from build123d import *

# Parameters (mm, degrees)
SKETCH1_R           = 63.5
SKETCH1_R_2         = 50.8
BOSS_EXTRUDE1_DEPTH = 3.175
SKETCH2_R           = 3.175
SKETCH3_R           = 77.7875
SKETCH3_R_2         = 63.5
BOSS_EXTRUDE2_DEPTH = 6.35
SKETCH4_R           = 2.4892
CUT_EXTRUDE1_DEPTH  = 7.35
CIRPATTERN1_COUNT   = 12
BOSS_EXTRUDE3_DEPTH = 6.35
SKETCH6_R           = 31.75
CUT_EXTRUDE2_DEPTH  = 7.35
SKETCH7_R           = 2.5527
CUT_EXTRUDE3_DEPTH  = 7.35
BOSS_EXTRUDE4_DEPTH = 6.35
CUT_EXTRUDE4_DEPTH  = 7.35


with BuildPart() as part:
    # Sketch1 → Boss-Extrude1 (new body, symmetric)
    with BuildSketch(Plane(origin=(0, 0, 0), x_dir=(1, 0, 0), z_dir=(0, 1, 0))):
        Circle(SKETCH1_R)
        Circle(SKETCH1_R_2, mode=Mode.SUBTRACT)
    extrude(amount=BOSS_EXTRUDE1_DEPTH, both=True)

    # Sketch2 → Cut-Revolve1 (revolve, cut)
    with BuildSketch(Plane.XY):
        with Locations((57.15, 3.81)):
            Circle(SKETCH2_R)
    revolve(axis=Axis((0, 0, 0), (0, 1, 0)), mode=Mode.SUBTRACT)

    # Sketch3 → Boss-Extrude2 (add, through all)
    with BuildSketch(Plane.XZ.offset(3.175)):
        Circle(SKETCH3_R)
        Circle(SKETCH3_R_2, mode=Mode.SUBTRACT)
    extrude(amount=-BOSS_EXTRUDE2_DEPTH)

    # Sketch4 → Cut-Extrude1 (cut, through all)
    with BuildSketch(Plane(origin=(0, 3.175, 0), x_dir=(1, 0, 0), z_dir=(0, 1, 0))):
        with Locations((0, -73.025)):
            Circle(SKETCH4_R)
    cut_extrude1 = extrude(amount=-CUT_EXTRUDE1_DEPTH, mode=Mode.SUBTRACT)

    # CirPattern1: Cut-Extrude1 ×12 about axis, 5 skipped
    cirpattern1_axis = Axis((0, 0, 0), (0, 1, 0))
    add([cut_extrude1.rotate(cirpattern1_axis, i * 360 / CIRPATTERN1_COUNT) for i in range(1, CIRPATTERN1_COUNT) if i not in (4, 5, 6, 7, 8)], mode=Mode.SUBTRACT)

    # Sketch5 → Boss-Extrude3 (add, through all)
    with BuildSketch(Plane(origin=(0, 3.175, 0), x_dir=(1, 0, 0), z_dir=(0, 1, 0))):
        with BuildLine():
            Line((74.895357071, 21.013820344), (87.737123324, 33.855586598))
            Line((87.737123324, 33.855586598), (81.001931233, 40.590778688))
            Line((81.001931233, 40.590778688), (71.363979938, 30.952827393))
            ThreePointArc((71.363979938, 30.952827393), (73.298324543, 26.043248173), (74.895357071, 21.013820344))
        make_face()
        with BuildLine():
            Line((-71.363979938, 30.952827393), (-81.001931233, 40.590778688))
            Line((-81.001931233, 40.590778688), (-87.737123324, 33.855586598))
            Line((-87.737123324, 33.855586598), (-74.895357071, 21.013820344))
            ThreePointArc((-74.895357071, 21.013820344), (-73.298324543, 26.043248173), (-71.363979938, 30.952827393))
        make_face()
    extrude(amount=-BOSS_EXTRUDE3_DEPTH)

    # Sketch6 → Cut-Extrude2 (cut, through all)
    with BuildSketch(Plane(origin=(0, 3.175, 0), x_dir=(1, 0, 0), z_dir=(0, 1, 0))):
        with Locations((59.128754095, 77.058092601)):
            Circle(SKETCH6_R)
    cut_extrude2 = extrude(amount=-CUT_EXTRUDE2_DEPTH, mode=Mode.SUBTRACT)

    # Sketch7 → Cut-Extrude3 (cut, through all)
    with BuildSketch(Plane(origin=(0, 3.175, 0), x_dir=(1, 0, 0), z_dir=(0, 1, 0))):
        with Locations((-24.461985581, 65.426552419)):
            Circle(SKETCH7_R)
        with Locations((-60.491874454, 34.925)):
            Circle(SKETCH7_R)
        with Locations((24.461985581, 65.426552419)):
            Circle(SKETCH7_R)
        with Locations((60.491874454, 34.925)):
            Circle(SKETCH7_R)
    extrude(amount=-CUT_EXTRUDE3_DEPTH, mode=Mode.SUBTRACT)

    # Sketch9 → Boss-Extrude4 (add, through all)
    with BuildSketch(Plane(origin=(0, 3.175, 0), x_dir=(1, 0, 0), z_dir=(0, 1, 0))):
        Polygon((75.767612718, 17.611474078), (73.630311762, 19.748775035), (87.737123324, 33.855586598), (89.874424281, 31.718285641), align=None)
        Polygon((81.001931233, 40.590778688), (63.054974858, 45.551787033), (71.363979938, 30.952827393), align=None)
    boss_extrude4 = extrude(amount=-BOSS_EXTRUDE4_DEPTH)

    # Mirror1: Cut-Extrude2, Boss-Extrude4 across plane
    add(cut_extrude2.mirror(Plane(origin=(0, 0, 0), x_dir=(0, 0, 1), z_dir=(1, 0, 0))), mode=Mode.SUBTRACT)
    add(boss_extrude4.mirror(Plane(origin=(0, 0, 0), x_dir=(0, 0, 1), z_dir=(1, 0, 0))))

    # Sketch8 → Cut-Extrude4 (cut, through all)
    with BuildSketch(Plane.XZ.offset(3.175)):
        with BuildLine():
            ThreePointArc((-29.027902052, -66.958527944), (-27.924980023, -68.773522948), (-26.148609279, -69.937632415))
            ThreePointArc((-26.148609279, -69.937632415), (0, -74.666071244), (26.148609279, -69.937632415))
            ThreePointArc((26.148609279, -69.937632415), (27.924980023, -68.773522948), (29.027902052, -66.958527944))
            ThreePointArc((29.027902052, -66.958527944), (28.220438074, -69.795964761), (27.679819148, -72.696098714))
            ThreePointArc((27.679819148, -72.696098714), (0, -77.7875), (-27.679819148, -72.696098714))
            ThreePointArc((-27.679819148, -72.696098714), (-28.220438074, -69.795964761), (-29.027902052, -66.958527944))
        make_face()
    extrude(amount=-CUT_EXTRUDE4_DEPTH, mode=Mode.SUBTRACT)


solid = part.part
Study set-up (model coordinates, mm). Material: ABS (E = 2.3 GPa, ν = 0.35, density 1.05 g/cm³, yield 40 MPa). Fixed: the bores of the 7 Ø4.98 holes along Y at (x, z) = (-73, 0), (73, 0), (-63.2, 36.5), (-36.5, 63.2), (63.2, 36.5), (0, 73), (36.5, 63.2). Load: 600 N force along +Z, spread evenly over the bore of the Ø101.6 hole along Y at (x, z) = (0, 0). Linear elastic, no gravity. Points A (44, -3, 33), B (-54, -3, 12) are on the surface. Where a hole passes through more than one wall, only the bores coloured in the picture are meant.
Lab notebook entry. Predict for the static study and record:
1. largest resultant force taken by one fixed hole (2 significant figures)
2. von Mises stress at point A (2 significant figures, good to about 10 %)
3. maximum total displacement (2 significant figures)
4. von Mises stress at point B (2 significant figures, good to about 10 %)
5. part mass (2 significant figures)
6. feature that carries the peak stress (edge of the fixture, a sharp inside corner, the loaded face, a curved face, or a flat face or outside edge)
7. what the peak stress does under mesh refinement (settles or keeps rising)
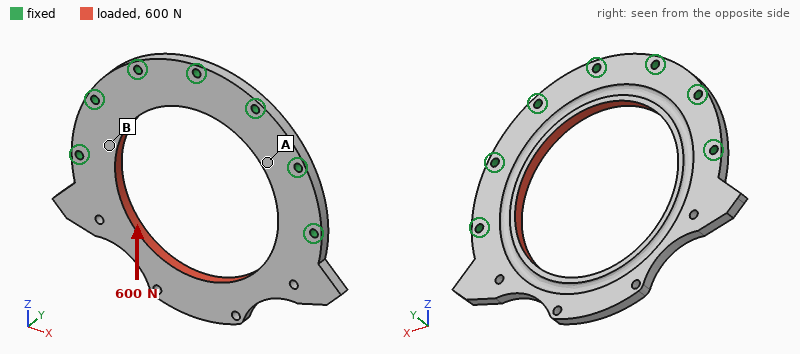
140 N
0.49 MPa
100 µm
1.0 MPa
65 g
edge of the fixture
keeps rising
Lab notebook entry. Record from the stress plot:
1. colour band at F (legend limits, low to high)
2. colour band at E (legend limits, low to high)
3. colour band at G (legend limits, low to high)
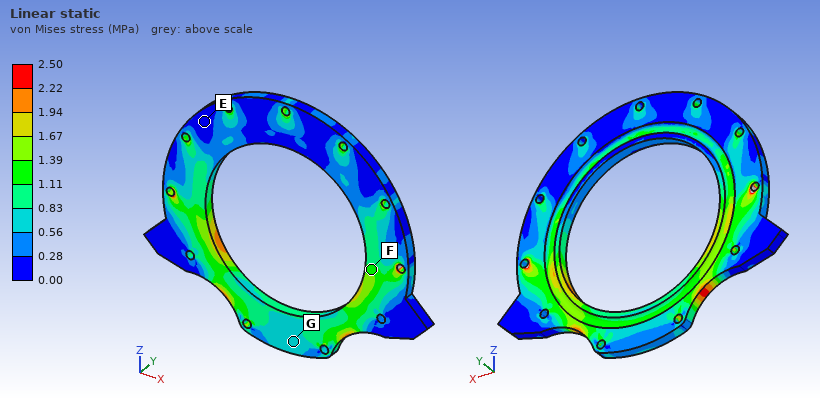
1.11 to 1.39 MPa
0.00 to 0.28 MPa
0.56 to 0.83 MPa
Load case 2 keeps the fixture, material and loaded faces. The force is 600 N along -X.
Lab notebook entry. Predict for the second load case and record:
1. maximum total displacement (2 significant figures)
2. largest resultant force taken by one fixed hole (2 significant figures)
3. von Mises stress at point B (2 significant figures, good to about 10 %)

0.20 mm
240 N
1.7 MPa
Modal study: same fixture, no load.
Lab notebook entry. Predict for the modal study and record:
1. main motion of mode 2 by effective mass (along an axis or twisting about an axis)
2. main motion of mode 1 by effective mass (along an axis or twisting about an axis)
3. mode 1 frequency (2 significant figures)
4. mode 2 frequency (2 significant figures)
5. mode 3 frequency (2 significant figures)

twisting about Z
along Y
200 Hz
540 Hz
850 Hz
